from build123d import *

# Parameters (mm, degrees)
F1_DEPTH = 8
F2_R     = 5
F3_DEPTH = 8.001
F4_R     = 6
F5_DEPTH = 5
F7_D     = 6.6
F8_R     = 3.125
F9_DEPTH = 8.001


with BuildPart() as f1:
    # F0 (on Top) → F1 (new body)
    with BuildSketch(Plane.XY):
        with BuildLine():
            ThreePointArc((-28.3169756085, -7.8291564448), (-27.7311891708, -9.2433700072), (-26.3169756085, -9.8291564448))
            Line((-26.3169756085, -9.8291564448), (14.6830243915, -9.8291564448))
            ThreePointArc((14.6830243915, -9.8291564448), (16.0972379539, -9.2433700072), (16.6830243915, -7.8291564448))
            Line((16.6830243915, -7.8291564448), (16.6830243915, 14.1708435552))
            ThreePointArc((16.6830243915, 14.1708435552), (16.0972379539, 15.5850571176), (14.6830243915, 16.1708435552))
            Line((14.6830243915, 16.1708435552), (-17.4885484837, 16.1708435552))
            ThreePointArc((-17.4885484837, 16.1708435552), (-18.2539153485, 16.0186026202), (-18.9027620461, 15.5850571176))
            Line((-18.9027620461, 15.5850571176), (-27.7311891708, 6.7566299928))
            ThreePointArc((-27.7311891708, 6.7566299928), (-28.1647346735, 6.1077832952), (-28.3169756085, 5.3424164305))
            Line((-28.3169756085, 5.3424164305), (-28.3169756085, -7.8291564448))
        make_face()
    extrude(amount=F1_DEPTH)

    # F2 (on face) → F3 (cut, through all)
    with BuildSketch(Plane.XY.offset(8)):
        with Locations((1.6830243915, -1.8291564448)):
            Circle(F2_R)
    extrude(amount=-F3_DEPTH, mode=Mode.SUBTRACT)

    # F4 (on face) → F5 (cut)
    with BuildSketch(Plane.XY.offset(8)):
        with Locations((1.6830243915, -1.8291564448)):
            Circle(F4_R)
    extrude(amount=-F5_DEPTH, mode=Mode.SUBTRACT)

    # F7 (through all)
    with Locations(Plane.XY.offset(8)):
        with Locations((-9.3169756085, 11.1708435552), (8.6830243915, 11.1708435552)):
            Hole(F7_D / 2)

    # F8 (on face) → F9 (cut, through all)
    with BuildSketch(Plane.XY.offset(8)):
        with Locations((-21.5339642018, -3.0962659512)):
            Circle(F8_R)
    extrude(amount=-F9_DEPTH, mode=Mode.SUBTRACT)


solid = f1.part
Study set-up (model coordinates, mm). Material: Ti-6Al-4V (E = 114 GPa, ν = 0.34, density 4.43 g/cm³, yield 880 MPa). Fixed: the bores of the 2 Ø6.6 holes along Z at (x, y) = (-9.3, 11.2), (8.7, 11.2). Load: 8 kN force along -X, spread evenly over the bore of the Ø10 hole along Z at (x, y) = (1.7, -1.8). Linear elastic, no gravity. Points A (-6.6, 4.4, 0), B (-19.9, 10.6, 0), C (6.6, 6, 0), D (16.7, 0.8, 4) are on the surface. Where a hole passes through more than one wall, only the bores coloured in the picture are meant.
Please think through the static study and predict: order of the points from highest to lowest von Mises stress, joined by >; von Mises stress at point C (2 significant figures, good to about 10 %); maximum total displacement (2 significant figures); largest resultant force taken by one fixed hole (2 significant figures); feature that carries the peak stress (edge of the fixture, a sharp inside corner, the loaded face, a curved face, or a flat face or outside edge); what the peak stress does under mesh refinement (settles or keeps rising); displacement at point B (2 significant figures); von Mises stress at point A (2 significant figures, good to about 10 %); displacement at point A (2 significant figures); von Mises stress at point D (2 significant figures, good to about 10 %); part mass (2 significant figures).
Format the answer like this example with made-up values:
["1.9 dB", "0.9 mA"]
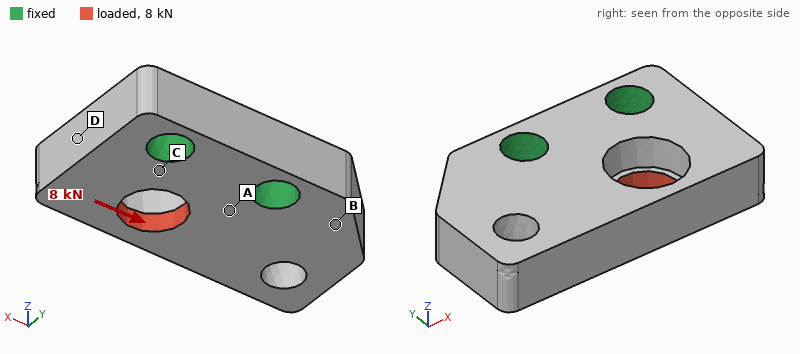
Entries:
["C > A > D > B", "100 MPa", "35 µm", "5.3 kN", "a sharp inside corner", "keeps rising", "8.1 µm", "84 MPa", "6.3 µm", "46 MPa", "33 g"]
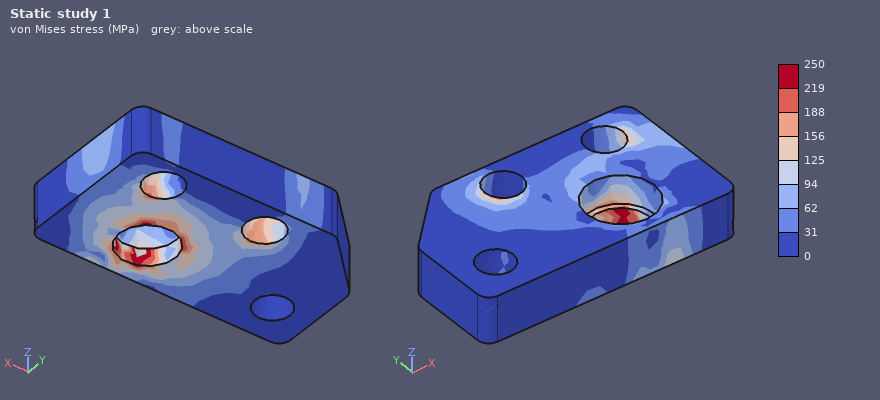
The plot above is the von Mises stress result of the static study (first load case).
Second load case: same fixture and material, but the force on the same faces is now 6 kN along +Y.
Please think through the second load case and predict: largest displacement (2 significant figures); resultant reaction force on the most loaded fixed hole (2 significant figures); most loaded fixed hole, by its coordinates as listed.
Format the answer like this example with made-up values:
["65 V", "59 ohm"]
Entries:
["26 µm", "3.6 kN", "(8.7, 11.2)"]
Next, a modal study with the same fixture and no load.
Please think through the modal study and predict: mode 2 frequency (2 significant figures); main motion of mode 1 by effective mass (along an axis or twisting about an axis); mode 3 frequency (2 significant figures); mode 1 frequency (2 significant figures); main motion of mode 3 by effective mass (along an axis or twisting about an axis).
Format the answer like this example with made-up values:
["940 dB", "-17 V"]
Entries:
["17 kHz", "along Z", "18 kHz", "12 kHz", "along X"]
